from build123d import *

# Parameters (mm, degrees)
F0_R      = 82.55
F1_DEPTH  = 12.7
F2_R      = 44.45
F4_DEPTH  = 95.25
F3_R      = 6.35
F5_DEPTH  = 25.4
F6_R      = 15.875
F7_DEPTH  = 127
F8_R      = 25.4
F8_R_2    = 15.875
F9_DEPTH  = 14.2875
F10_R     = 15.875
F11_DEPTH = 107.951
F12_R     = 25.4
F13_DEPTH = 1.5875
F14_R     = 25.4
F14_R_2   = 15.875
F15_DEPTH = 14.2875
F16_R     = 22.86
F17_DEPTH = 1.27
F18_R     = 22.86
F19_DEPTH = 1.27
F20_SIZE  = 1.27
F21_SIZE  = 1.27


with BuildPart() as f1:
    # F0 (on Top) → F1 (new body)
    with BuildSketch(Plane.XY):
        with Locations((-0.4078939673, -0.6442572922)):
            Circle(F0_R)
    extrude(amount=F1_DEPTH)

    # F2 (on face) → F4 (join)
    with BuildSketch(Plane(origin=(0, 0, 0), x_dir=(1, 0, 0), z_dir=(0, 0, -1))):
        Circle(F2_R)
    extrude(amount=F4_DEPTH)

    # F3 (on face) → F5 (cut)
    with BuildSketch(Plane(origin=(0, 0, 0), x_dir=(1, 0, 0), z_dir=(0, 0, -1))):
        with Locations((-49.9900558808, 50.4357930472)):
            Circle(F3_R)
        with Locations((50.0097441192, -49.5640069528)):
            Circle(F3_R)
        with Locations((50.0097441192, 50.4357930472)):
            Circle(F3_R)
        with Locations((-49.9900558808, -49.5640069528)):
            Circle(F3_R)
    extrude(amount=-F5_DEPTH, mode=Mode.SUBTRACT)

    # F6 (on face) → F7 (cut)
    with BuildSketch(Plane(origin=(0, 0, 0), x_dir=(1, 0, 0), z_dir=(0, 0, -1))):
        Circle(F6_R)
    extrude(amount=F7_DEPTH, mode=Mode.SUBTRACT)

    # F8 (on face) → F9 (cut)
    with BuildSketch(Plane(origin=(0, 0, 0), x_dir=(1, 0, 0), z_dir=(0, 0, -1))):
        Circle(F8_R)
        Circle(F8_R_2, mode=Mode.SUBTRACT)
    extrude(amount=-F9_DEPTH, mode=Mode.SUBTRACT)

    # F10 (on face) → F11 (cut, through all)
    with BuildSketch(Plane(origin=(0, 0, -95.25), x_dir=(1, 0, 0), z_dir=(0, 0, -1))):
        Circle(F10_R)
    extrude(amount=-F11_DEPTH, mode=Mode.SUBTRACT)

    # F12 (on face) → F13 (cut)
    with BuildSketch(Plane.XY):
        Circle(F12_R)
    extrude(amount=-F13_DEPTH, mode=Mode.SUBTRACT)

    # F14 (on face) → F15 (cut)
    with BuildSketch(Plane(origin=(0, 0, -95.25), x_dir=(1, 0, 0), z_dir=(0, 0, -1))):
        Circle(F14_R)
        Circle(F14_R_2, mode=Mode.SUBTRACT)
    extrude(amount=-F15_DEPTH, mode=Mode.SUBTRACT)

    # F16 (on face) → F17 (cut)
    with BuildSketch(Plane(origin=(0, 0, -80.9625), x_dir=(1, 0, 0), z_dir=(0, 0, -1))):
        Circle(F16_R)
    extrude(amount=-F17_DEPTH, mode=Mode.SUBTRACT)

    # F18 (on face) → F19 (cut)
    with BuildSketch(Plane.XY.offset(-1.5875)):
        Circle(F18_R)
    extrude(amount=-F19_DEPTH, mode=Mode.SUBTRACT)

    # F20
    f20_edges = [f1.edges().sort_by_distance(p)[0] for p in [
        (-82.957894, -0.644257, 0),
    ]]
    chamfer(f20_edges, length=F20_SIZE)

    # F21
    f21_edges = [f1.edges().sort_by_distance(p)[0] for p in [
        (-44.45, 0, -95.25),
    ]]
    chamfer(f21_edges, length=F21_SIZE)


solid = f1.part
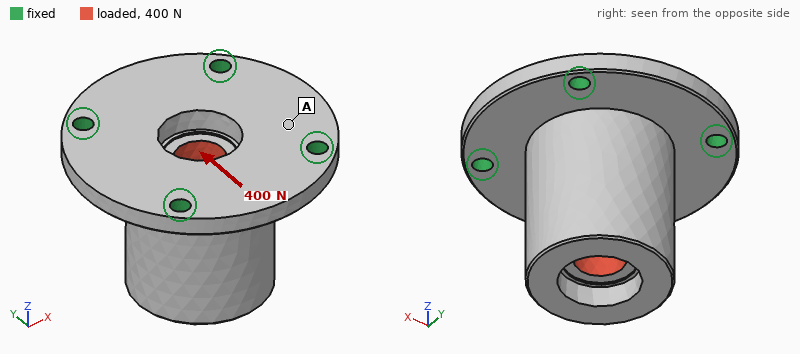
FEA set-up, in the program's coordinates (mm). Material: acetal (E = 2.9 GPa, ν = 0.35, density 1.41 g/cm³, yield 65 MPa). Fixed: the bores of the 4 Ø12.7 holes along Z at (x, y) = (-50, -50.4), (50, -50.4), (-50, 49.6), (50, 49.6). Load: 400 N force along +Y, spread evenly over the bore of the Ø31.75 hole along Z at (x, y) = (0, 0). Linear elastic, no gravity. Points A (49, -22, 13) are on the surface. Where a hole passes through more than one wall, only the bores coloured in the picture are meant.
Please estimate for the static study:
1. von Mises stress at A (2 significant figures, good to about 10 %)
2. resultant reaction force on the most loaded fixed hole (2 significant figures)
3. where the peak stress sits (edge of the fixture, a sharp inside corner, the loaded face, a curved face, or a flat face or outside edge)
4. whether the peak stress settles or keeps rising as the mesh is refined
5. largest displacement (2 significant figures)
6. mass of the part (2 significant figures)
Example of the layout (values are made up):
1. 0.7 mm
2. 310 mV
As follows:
1. 0.22 MPa
2. 150 N
3. edge of the fixture
4. keeps rising
5. 53 µm
6. 1.0 kg
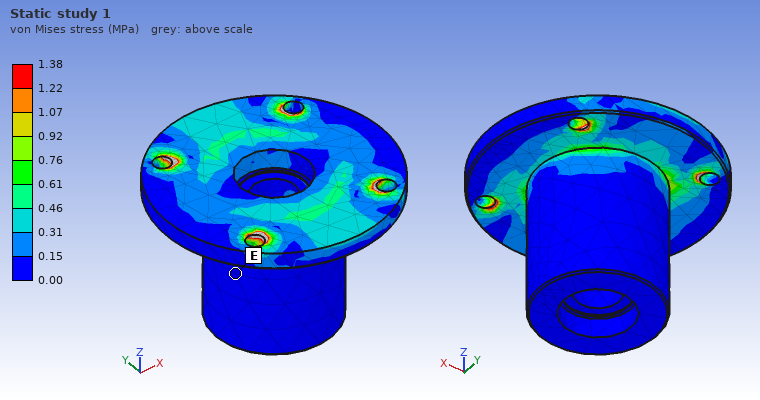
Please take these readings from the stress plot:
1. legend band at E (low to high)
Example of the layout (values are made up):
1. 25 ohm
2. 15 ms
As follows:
1. 0.00 to 0.15 MPa
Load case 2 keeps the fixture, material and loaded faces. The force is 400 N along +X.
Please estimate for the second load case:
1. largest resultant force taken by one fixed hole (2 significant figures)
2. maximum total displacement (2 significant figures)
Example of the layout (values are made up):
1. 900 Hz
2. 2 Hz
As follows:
1. 150 N
2. 53 µm
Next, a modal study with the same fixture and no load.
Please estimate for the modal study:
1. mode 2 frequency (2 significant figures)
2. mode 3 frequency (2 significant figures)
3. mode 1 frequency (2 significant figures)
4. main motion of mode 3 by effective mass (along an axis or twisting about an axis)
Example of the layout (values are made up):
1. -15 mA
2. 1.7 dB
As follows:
1. 580 Hz
2. 870 Hz
3. 580 Hz
4. along Z
